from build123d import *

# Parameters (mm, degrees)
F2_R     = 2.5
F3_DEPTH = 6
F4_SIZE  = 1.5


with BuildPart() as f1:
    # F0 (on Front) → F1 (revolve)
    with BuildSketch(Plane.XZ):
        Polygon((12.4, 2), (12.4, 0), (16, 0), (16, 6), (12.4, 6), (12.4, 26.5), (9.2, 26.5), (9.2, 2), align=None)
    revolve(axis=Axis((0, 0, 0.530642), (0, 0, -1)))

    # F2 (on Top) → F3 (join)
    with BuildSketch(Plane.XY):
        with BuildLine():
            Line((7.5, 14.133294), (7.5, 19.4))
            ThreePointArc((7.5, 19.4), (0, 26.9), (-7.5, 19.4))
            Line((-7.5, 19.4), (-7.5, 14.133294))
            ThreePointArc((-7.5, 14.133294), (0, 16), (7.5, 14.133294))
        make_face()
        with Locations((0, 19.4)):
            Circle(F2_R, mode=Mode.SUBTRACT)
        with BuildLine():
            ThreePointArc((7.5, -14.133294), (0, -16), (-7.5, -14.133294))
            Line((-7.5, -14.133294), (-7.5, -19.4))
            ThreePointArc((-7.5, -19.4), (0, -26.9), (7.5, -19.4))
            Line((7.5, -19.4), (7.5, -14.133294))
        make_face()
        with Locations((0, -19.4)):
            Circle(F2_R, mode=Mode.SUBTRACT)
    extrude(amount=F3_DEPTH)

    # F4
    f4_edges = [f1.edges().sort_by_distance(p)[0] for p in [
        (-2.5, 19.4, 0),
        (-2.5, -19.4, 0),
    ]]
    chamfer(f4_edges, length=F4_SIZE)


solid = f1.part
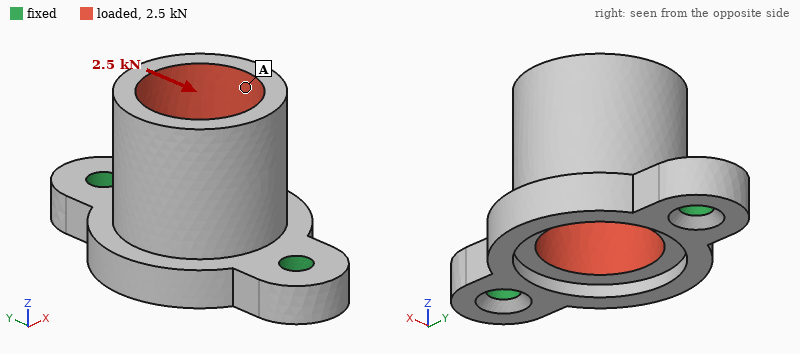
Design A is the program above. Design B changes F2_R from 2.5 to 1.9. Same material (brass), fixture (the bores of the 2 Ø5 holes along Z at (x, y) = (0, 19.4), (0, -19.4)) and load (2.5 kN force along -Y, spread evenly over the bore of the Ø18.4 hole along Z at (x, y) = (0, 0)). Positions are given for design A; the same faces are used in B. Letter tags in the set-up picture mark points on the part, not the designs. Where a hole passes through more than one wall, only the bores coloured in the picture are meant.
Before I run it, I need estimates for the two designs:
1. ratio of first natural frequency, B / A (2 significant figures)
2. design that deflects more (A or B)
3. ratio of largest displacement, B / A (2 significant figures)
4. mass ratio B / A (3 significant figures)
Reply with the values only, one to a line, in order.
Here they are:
0.93
B
1.1
1.01
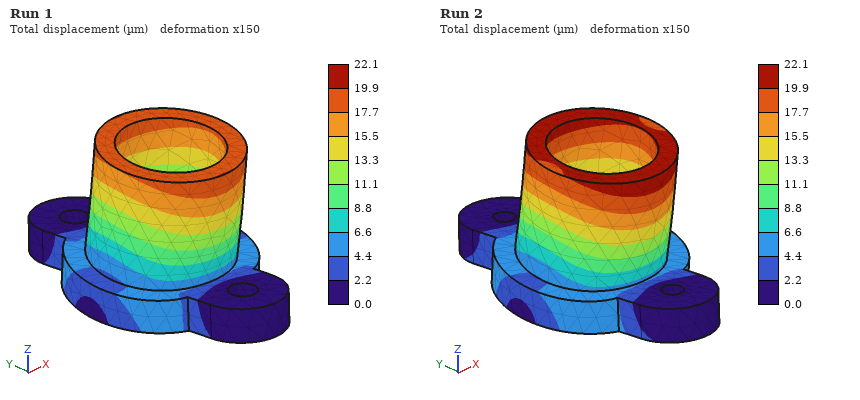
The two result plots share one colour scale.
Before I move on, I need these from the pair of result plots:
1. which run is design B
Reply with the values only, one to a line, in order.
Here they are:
Run 2
